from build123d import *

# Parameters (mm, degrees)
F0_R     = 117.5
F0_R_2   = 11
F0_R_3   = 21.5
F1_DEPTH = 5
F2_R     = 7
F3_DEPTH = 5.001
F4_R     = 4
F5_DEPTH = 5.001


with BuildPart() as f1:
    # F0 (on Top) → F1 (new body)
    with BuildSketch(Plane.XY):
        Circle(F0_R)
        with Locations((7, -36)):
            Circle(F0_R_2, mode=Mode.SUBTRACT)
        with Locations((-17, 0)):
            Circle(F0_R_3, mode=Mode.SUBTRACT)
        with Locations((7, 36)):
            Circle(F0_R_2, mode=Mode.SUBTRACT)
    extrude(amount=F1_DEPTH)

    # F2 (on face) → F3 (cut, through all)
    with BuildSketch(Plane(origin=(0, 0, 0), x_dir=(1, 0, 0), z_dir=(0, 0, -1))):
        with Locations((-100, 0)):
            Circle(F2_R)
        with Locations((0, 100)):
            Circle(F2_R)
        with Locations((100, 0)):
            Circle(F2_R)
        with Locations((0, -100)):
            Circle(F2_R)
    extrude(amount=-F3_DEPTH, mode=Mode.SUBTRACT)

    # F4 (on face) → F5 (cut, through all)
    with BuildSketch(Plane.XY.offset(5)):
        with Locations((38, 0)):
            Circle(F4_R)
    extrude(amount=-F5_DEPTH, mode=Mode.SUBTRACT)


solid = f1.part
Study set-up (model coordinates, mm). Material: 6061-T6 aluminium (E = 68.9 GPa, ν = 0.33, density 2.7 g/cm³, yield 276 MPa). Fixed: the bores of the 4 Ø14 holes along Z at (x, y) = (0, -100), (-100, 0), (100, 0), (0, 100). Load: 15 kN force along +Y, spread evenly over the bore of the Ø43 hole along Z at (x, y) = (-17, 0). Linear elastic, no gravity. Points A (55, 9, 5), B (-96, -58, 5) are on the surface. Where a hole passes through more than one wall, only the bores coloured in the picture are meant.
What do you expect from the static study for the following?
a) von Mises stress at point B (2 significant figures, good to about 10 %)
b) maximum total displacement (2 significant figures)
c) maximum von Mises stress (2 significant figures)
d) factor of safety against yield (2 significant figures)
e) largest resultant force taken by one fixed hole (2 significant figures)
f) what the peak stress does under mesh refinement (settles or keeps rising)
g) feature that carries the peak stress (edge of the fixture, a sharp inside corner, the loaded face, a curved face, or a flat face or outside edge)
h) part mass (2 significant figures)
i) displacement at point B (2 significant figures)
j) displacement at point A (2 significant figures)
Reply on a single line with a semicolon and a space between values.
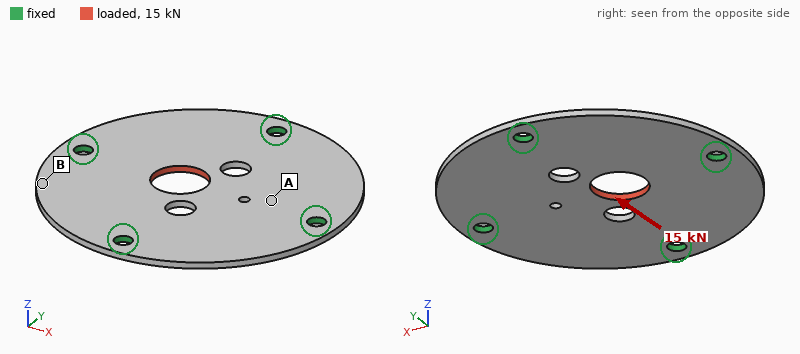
9.2 MPa; 35 µm; 70 MPa; 3.9; 4.6 kN; settles; a curved face; 550 g; 12 µm; 9.5 µm
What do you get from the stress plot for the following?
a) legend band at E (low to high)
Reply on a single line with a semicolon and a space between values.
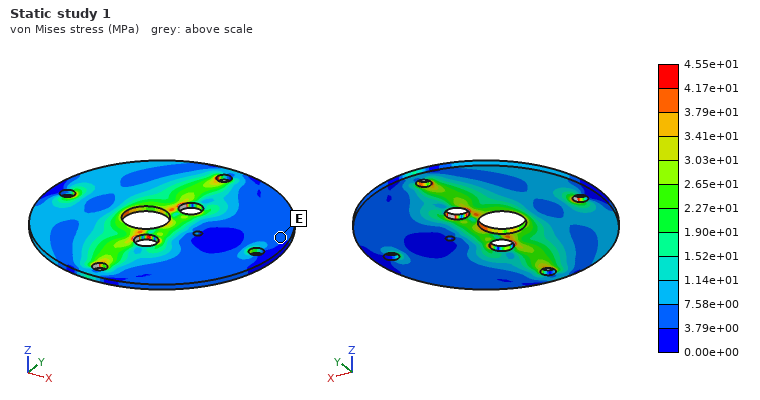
3.79e+00 to 7.58e+00 MPa
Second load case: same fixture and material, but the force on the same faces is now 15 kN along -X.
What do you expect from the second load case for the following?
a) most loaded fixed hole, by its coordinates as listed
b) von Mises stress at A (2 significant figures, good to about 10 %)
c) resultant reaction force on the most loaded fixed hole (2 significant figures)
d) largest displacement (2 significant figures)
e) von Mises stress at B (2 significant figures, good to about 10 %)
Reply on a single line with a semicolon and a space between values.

(-100, 0); 19 MPa; 5.8 kN; 30 µm; 7.9 MPa
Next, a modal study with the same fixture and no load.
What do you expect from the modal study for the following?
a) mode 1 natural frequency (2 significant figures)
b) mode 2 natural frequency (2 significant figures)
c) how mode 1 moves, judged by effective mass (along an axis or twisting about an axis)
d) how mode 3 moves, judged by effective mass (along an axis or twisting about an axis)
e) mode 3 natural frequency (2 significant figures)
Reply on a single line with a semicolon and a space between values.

1000 Hz; 1100 Hz; along Z; twisting about X; 1200 Hz
